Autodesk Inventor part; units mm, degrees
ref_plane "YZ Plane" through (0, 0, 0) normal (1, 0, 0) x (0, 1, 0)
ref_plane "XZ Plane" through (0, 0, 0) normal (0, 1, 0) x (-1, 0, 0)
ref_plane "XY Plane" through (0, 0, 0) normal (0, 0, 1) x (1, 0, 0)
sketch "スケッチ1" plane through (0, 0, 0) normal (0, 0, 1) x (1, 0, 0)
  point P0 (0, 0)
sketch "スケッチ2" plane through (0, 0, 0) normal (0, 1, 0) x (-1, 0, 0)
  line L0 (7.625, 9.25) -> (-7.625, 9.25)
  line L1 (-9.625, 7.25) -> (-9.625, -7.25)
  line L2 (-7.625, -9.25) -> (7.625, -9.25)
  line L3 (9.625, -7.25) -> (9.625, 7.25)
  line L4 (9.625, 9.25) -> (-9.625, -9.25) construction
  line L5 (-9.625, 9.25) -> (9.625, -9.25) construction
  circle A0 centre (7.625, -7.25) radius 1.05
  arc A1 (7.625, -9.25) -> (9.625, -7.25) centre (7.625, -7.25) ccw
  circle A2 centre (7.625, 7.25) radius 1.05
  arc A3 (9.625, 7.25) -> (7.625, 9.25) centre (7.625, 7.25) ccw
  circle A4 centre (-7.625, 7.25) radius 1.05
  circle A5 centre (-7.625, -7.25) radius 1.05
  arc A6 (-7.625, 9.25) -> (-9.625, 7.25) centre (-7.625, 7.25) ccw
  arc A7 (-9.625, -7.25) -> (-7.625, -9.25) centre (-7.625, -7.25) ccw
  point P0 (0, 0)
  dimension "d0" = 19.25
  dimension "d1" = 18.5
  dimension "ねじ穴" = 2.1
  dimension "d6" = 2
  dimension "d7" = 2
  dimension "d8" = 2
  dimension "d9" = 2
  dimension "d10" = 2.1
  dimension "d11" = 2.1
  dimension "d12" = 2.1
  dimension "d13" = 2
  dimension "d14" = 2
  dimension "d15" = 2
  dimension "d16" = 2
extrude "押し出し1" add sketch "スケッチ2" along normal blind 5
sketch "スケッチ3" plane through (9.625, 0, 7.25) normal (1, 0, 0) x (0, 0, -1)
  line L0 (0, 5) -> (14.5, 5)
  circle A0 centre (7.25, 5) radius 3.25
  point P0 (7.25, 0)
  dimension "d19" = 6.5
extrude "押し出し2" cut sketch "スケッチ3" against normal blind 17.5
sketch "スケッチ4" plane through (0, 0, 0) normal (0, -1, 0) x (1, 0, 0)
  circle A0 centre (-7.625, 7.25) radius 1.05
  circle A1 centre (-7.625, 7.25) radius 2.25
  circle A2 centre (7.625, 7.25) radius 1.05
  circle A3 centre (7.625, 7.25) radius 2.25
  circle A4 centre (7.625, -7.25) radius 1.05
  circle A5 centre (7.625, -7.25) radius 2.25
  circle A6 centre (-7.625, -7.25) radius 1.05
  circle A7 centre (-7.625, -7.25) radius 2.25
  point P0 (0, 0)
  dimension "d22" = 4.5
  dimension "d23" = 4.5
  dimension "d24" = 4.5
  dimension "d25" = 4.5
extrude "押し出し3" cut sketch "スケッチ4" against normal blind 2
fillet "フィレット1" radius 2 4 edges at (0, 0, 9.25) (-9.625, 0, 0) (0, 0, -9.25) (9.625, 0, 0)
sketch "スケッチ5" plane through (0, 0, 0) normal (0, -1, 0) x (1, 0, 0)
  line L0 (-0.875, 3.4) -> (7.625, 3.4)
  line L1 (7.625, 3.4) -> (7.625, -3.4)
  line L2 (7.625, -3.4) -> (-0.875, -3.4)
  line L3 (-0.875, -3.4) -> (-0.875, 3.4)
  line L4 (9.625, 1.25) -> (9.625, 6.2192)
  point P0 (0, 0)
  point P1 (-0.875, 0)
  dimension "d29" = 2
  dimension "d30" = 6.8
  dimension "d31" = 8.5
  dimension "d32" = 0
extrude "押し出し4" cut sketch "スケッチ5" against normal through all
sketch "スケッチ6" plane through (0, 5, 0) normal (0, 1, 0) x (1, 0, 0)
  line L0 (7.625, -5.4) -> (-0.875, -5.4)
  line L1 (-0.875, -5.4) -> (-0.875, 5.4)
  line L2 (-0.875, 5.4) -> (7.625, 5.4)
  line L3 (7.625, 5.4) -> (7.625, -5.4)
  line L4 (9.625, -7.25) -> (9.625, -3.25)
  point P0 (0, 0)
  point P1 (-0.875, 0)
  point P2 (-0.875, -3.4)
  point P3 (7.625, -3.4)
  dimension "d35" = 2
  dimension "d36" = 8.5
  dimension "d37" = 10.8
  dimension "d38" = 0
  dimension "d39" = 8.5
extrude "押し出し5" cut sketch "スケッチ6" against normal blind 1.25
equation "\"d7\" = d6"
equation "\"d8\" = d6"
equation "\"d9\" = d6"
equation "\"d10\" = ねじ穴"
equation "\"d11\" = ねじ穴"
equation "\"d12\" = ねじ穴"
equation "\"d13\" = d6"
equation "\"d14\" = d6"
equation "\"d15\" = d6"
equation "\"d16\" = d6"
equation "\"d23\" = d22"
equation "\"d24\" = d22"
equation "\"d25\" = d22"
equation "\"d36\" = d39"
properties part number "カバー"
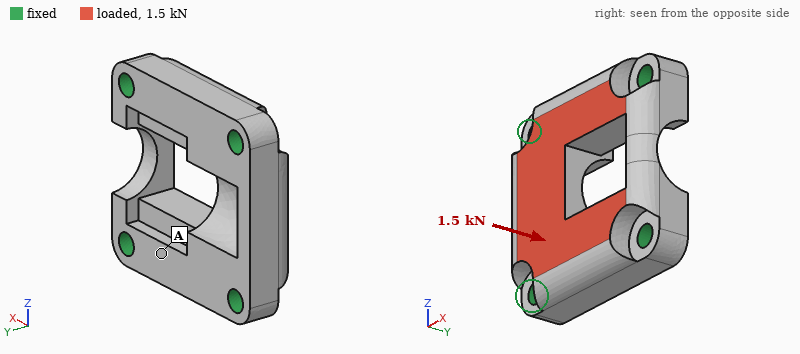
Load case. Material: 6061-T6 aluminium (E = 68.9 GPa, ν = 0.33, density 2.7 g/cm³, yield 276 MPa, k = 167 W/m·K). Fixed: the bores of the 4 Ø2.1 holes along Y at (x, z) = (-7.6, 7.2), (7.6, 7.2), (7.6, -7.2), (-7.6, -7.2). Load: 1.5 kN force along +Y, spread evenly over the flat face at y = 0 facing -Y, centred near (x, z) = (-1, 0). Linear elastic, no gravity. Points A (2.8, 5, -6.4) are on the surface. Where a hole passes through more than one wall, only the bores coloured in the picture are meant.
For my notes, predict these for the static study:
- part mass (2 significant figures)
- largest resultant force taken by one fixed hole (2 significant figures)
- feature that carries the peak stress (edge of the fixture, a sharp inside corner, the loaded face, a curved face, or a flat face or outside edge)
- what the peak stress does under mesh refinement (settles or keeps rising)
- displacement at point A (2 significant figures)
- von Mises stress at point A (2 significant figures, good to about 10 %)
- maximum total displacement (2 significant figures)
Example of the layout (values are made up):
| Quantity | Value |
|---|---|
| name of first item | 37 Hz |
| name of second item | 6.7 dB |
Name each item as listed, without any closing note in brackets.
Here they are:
| Quantity | Value |
|---|---|
| part mass | 2.9 g |
| largest resultant force taken by one fixed hole | 570 N |
| feature that carries the peak stress | edge of the fixture |
| what the peak stress does under mesh refinement | keeps rising |
| displacement at point A | 5.6 µm |
| von Mises stress at point A | 21 MPa |
| maximum total displacement | 14 µm |
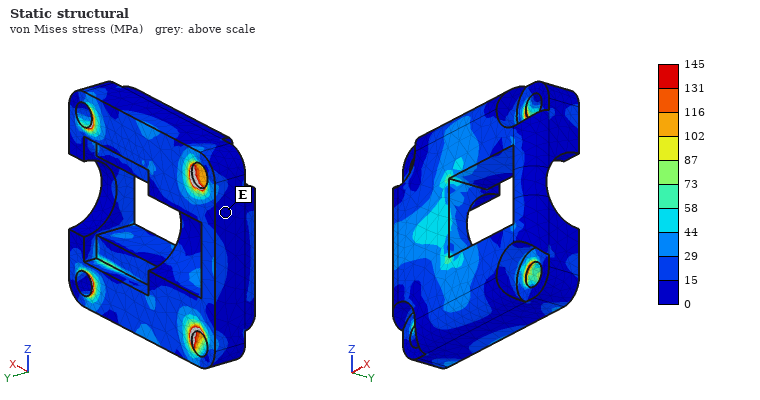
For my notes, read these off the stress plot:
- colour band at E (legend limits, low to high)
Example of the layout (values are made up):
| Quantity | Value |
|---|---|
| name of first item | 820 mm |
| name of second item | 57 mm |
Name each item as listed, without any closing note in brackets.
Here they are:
| Quantity | Value |
|---|---|
| colour band at E | 0 to 15 MPa |
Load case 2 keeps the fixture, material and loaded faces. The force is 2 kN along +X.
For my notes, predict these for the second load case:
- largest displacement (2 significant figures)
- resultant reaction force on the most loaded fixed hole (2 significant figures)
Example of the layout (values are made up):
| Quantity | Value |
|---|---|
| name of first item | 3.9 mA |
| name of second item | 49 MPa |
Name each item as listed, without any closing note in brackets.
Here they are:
| Quantity | Value |
|---|---|
| largest displacement | 11 µm |
| resultant reaction force on the most loaded fixed hole | 570 N |
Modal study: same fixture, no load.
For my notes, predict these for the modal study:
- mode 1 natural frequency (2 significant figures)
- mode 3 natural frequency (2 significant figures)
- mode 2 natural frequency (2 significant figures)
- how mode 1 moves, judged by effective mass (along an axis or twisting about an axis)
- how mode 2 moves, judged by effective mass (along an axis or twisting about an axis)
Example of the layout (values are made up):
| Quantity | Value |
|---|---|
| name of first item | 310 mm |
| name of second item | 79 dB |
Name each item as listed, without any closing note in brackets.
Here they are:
| Quantity | Value |
|---|---|
| mode 1 natural frequency | 54 kHz |
| mode 3 natural frequency | 68 kHz |
| mode 2 natural frequency | 60 kHz |
| how mode 1 moves, judged by effective mass | along Y |
| how mode 2 moves, judged by effective mass | along Z |
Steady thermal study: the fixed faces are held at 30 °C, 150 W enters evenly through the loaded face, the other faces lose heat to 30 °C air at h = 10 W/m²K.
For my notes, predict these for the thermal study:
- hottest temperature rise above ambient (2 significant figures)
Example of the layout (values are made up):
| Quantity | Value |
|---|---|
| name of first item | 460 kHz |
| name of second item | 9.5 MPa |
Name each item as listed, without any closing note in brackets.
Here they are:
| Quantity | Value |
|---|---|
| hottest temperature rise above ambient | 70 K |
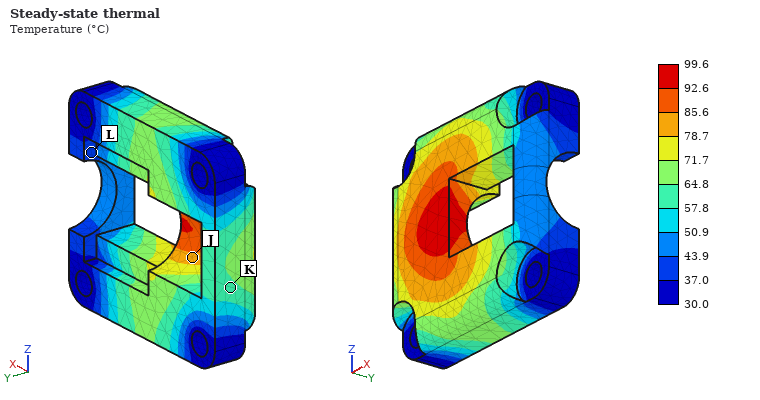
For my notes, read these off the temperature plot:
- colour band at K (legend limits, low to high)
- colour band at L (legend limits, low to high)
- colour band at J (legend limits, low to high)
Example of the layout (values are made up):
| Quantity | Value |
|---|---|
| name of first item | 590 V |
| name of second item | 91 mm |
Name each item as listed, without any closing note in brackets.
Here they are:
| Quantity | Value |
|---|---|
| colour band at K | 57.8 to 64.8 °C |
| colour band at L | 37.0 to 43.9 °C |
| colour band at J | 78.7 to 85.6 °C |
